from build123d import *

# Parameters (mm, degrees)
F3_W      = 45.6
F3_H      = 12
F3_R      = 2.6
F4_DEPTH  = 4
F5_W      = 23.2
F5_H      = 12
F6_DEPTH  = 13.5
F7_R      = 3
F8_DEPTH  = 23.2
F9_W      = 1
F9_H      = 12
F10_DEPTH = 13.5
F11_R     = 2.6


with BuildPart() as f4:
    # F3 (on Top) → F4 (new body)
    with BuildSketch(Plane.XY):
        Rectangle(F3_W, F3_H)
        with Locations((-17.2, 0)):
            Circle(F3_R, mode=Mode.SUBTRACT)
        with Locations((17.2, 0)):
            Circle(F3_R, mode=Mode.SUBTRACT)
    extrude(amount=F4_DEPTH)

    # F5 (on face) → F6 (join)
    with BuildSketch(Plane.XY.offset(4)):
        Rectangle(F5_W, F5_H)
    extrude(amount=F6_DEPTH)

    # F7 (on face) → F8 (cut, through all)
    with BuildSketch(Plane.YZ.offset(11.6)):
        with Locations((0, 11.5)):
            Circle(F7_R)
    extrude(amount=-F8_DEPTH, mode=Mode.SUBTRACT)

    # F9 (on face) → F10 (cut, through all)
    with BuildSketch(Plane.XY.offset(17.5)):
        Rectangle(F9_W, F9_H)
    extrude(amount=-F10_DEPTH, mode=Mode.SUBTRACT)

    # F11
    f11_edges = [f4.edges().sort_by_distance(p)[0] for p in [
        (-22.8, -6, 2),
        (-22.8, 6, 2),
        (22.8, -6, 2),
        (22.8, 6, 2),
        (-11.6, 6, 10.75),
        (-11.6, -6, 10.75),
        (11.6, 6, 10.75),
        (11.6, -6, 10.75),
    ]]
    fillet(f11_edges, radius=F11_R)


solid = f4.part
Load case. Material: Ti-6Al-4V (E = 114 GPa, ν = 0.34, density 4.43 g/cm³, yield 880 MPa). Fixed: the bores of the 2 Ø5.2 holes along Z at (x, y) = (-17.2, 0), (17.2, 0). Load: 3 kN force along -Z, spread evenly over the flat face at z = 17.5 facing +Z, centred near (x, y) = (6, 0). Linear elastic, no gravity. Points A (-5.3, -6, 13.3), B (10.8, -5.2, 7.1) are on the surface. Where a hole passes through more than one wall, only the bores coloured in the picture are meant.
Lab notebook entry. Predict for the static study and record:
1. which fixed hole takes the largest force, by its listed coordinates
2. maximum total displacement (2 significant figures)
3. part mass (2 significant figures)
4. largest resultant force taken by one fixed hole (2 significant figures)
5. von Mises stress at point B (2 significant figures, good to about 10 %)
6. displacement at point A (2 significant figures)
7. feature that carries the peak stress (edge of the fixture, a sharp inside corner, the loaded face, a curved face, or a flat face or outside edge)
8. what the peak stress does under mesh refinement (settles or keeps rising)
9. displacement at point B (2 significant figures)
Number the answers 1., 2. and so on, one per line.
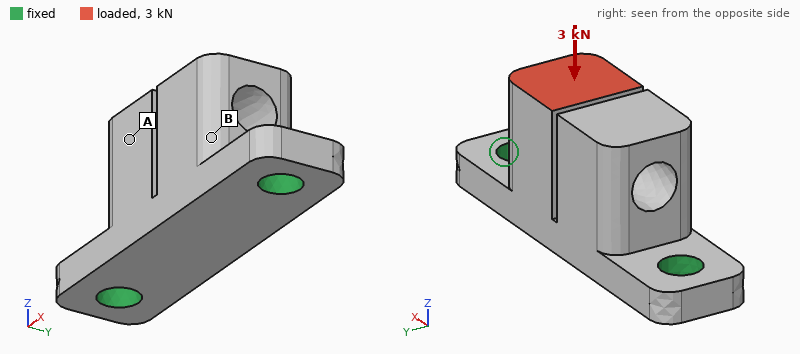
1. (17.2, 0)
2. 58 µm
3. 22 g
4. 2.3 kN
5. 56 MPa
6. 37 µm
7. edge of the fixture
8. keeps rising
9. 21 µm
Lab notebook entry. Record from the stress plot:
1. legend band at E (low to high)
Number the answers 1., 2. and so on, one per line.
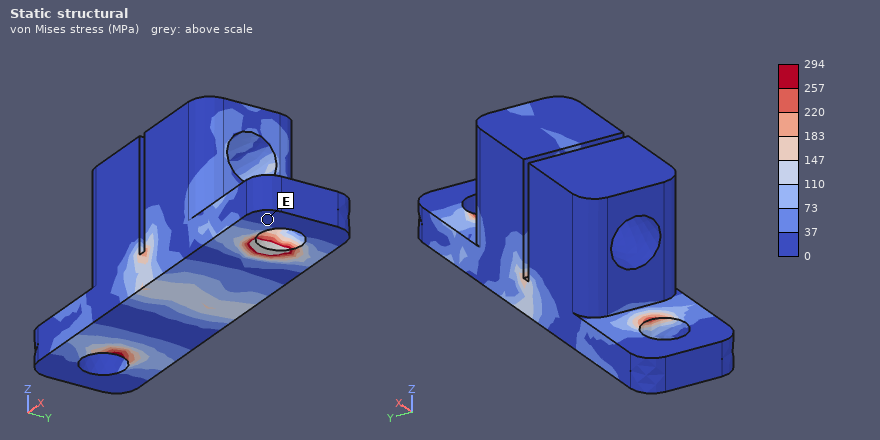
1. 0 to 37 MPa
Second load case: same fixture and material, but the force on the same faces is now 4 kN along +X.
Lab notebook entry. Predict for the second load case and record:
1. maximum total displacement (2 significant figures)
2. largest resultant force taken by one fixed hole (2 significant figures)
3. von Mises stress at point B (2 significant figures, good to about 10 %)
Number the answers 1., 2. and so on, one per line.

1. 0.21 mm
2. 3.1 kN
3. 240 MPa
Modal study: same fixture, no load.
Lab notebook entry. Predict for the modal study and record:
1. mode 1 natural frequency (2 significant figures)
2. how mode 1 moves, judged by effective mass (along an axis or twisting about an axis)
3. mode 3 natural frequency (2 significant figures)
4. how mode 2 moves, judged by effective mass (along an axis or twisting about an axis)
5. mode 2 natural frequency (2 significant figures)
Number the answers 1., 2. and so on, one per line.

1. 8200 Hz
2. along Y
3. 16 kHz
4. along Z
5. 9400 Hz
